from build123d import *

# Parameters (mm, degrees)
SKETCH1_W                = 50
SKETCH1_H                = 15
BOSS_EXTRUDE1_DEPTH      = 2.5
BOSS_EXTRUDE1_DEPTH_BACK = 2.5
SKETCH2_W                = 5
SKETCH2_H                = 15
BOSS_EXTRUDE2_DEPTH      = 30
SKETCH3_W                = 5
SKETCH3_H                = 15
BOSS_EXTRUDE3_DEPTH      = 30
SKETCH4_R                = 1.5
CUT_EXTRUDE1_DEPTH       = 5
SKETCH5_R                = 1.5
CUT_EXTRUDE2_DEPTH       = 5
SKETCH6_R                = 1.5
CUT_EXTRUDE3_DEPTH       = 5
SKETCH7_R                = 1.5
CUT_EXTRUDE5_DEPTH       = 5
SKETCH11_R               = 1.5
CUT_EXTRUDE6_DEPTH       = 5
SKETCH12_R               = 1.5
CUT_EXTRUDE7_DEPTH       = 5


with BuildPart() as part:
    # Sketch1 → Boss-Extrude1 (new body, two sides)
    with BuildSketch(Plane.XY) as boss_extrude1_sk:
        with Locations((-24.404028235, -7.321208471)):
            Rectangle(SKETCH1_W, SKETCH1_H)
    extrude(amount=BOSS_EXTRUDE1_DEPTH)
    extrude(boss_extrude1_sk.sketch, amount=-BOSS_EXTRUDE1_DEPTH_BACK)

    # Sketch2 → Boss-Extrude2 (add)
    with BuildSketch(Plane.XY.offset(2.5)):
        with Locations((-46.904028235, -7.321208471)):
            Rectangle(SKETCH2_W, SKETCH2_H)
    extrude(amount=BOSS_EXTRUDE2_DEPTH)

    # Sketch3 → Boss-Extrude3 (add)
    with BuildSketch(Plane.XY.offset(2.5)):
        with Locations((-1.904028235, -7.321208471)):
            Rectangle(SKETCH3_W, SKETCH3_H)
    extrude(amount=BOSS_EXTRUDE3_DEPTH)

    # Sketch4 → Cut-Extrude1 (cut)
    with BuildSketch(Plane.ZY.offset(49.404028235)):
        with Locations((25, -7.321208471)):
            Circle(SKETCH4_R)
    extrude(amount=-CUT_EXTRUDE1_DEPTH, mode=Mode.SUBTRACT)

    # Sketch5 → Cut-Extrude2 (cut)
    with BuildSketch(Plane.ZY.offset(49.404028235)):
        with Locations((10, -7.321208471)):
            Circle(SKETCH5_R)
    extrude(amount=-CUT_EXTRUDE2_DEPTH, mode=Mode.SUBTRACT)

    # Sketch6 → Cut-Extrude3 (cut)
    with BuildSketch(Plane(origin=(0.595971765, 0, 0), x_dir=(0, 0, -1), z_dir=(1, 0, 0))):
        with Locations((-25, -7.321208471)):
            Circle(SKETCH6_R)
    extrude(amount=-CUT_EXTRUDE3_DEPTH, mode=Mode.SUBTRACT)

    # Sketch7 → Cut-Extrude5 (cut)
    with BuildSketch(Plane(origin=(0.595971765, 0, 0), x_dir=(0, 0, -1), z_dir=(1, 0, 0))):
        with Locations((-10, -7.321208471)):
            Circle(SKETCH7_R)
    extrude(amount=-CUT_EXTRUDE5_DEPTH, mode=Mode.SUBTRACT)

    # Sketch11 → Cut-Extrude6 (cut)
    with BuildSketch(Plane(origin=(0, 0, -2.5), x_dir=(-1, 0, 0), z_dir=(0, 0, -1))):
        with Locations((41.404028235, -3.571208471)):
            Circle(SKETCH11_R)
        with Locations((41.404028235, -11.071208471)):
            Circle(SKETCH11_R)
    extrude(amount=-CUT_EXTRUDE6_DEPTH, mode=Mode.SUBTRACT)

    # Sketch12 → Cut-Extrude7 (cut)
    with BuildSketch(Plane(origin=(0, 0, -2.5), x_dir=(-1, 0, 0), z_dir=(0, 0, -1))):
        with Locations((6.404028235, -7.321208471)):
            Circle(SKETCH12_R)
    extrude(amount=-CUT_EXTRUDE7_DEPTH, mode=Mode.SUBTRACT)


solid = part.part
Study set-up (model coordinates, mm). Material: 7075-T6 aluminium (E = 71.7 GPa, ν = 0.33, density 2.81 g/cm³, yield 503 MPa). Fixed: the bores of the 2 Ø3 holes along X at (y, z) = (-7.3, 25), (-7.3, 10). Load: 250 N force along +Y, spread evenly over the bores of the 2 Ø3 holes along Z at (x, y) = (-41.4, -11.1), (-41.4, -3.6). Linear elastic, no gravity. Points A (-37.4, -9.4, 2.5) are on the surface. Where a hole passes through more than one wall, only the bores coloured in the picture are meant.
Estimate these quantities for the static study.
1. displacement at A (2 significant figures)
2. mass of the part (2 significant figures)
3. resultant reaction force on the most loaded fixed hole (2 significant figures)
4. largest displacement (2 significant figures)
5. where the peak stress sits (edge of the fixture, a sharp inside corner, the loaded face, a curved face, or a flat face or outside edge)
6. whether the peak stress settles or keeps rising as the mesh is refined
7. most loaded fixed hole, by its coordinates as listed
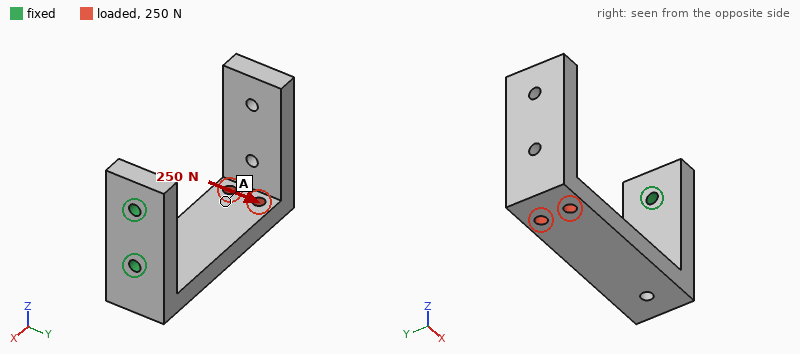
0.26 mm
22 g
360 N
0.39 mm
edge of the fixture
keeps rising
(-7.3, 10)
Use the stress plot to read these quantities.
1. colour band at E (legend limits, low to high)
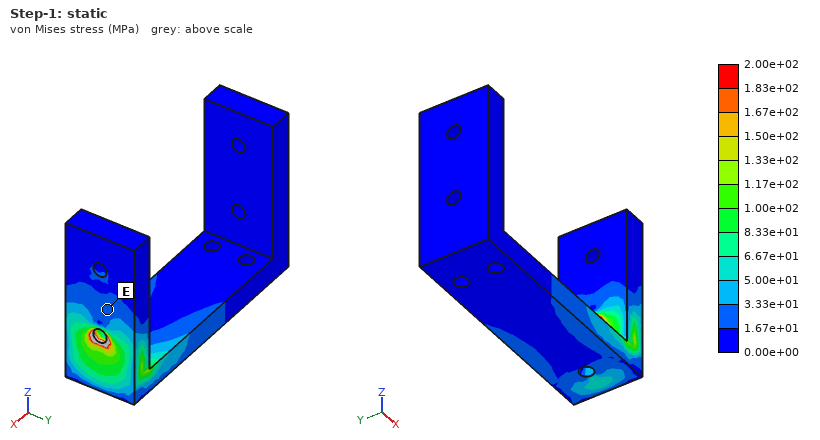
1.67e+01 to 3.33e+01 MPa
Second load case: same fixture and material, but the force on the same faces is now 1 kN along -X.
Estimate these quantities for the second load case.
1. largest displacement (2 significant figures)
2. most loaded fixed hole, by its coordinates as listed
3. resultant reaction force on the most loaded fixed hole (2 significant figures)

0.26 mm
(-7.3, 10)
1.2 kN
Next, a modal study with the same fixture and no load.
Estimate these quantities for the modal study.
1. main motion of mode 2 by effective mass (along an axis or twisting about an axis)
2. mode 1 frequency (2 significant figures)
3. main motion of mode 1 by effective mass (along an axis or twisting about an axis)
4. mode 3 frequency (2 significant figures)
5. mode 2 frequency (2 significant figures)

along Y
720 Hz
along Z
2300 Hz
1100 Hz
